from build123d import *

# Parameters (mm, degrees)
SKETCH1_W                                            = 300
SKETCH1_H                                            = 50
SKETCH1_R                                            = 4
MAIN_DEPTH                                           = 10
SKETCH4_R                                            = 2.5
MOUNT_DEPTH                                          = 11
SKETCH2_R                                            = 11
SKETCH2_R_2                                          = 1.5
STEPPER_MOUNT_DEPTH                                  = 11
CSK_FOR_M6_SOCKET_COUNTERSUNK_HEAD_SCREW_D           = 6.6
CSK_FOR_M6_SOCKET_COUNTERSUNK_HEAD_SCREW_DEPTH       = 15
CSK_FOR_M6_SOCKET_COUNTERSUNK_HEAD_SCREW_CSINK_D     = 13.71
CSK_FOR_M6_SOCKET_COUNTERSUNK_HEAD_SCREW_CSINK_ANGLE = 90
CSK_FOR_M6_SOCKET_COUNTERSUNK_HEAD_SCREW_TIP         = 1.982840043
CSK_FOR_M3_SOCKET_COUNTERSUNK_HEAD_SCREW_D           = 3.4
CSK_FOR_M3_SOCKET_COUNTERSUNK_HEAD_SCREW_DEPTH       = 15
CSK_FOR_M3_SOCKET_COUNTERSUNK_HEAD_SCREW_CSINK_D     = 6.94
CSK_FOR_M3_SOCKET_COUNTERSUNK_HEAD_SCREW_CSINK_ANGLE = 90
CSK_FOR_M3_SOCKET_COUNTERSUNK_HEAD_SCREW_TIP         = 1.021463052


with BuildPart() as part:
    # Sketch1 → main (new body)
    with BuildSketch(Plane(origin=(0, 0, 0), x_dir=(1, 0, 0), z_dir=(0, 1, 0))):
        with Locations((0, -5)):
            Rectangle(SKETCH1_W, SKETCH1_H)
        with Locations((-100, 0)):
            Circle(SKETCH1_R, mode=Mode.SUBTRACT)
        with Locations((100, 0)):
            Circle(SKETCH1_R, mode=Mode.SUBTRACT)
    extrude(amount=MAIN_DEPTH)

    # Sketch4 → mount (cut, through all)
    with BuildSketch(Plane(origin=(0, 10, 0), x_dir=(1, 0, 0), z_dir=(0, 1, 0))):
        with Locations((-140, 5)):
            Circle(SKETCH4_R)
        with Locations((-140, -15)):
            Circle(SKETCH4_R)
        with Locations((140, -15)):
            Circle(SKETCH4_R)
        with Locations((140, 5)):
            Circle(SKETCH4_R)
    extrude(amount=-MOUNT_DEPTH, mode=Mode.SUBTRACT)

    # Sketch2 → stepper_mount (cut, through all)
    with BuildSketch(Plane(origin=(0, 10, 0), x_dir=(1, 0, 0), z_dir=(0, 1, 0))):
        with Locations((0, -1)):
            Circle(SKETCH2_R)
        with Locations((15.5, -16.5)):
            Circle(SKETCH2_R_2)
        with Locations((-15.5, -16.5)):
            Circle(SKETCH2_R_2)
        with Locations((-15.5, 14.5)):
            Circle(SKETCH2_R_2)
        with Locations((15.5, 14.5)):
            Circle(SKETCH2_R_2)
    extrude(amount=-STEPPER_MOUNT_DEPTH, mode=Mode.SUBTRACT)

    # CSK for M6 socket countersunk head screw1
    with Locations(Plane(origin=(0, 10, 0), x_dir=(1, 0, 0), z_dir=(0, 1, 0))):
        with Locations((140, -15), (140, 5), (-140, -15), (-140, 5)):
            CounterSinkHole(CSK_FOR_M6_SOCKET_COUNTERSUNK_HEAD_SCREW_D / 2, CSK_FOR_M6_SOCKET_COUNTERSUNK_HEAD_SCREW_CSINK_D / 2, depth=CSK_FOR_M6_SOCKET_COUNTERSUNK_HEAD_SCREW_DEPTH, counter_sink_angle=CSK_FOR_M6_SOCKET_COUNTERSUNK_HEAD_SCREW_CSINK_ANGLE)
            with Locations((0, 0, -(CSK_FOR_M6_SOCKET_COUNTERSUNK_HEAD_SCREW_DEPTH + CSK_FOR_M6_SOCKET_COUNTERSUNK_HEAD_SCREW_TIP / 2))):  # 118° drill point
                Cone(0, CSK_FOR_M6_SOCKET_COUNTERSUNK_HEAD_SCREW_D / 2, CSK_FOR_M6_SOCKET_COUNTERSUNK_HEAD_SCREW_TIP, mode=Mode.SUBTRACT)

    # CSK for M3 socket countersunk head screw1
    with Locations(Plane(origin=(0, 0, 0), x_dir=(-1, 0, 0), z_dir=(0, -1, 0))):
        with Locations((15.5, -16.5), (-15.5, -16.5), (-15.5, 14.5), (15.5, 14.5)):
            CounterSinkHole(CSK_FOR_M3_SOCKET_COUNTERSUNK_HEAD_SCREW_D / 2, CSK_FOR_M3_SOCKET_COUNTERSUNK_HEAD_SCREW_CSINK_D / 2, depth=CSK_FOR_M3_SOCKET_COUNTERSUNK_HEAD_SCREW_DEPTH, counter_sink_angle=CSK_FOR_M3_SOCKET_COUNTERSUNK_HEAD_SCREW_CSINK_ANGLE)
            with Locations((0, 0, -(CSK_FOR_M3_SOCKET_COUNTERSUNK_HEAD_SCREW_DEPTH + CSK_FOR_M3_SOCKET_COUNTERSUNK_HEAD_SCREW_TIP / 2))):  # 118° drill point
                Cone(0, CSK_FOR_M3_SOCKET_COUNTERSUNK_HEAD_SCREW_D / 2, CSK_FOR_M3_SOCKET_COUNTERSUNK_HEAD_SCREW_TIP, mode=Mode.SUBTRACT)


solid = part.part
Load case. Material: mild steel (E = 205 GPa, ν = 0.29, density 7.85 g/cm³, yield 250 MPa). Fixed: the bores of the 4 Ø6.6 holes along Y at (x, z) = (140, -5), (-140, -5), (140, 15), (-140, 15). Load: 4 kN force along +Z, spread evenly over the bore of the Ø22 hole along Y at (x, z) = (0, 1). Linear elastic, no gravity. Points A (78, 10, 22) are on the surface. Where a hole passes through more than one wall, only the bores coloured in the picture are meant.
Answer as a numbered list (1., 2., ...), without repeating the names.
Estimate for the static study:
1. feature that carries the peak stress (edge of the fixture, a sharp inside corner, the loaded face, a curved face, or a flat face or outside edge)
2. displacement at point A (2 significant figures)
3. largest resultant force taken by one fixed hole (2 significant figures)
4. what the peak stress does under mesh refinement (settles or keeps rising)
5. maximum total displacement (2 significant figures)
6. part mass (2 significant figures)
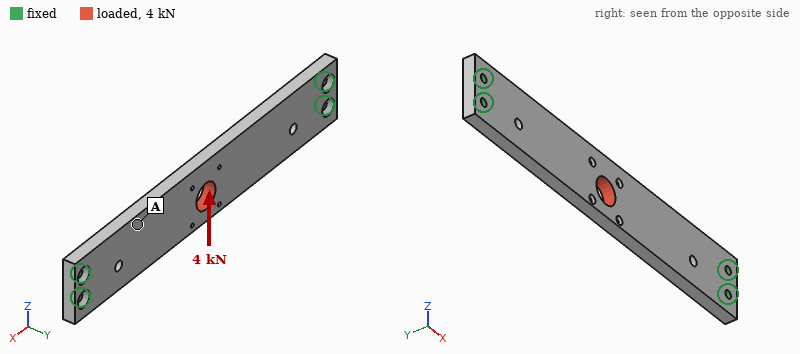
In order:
1. edge of the fixture
2. 19 µm
3. 5.1 kN
4. keeps rising
5. 40 µm
6. 1.1 kg
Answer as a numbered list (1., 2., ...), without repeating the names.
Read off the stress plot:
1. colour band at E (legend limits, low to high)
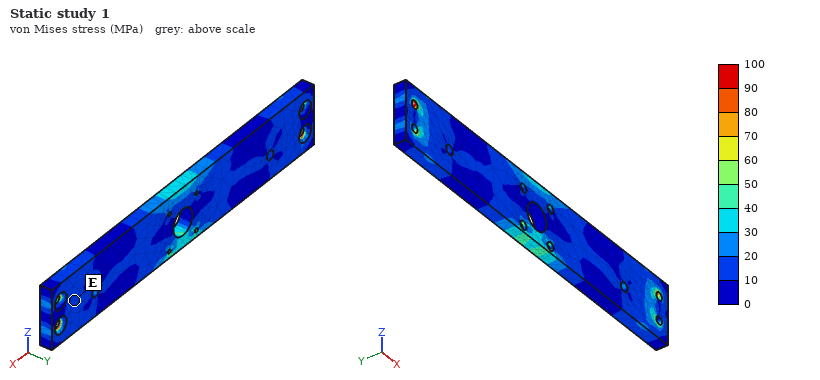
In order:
1. 10 to 20 MPa
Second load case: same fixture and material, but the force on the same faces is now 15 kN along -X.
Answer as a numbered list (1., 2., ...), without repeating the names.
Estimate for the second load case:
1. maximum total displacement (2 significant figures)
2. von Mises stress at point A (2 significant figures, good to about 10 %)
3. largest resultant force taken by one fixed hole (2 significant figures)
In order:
1. 13 µm
2. 13 MPa
3. 4.1 kN
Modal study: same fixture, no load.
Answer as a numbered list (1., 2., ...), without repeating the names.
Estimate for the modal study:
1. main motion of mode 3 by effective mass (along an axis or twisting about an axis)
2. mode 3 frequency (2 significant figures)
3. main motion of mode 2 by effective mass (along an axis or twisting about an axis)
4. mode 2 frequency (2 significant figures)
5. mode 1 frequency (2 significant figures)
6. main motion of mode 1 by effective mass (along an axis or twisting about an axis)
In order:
1. twisting about X
2. 2200 Hz
3. twisting about Z
4. 1700 Hz
5. 620 Hz
6. along Y
